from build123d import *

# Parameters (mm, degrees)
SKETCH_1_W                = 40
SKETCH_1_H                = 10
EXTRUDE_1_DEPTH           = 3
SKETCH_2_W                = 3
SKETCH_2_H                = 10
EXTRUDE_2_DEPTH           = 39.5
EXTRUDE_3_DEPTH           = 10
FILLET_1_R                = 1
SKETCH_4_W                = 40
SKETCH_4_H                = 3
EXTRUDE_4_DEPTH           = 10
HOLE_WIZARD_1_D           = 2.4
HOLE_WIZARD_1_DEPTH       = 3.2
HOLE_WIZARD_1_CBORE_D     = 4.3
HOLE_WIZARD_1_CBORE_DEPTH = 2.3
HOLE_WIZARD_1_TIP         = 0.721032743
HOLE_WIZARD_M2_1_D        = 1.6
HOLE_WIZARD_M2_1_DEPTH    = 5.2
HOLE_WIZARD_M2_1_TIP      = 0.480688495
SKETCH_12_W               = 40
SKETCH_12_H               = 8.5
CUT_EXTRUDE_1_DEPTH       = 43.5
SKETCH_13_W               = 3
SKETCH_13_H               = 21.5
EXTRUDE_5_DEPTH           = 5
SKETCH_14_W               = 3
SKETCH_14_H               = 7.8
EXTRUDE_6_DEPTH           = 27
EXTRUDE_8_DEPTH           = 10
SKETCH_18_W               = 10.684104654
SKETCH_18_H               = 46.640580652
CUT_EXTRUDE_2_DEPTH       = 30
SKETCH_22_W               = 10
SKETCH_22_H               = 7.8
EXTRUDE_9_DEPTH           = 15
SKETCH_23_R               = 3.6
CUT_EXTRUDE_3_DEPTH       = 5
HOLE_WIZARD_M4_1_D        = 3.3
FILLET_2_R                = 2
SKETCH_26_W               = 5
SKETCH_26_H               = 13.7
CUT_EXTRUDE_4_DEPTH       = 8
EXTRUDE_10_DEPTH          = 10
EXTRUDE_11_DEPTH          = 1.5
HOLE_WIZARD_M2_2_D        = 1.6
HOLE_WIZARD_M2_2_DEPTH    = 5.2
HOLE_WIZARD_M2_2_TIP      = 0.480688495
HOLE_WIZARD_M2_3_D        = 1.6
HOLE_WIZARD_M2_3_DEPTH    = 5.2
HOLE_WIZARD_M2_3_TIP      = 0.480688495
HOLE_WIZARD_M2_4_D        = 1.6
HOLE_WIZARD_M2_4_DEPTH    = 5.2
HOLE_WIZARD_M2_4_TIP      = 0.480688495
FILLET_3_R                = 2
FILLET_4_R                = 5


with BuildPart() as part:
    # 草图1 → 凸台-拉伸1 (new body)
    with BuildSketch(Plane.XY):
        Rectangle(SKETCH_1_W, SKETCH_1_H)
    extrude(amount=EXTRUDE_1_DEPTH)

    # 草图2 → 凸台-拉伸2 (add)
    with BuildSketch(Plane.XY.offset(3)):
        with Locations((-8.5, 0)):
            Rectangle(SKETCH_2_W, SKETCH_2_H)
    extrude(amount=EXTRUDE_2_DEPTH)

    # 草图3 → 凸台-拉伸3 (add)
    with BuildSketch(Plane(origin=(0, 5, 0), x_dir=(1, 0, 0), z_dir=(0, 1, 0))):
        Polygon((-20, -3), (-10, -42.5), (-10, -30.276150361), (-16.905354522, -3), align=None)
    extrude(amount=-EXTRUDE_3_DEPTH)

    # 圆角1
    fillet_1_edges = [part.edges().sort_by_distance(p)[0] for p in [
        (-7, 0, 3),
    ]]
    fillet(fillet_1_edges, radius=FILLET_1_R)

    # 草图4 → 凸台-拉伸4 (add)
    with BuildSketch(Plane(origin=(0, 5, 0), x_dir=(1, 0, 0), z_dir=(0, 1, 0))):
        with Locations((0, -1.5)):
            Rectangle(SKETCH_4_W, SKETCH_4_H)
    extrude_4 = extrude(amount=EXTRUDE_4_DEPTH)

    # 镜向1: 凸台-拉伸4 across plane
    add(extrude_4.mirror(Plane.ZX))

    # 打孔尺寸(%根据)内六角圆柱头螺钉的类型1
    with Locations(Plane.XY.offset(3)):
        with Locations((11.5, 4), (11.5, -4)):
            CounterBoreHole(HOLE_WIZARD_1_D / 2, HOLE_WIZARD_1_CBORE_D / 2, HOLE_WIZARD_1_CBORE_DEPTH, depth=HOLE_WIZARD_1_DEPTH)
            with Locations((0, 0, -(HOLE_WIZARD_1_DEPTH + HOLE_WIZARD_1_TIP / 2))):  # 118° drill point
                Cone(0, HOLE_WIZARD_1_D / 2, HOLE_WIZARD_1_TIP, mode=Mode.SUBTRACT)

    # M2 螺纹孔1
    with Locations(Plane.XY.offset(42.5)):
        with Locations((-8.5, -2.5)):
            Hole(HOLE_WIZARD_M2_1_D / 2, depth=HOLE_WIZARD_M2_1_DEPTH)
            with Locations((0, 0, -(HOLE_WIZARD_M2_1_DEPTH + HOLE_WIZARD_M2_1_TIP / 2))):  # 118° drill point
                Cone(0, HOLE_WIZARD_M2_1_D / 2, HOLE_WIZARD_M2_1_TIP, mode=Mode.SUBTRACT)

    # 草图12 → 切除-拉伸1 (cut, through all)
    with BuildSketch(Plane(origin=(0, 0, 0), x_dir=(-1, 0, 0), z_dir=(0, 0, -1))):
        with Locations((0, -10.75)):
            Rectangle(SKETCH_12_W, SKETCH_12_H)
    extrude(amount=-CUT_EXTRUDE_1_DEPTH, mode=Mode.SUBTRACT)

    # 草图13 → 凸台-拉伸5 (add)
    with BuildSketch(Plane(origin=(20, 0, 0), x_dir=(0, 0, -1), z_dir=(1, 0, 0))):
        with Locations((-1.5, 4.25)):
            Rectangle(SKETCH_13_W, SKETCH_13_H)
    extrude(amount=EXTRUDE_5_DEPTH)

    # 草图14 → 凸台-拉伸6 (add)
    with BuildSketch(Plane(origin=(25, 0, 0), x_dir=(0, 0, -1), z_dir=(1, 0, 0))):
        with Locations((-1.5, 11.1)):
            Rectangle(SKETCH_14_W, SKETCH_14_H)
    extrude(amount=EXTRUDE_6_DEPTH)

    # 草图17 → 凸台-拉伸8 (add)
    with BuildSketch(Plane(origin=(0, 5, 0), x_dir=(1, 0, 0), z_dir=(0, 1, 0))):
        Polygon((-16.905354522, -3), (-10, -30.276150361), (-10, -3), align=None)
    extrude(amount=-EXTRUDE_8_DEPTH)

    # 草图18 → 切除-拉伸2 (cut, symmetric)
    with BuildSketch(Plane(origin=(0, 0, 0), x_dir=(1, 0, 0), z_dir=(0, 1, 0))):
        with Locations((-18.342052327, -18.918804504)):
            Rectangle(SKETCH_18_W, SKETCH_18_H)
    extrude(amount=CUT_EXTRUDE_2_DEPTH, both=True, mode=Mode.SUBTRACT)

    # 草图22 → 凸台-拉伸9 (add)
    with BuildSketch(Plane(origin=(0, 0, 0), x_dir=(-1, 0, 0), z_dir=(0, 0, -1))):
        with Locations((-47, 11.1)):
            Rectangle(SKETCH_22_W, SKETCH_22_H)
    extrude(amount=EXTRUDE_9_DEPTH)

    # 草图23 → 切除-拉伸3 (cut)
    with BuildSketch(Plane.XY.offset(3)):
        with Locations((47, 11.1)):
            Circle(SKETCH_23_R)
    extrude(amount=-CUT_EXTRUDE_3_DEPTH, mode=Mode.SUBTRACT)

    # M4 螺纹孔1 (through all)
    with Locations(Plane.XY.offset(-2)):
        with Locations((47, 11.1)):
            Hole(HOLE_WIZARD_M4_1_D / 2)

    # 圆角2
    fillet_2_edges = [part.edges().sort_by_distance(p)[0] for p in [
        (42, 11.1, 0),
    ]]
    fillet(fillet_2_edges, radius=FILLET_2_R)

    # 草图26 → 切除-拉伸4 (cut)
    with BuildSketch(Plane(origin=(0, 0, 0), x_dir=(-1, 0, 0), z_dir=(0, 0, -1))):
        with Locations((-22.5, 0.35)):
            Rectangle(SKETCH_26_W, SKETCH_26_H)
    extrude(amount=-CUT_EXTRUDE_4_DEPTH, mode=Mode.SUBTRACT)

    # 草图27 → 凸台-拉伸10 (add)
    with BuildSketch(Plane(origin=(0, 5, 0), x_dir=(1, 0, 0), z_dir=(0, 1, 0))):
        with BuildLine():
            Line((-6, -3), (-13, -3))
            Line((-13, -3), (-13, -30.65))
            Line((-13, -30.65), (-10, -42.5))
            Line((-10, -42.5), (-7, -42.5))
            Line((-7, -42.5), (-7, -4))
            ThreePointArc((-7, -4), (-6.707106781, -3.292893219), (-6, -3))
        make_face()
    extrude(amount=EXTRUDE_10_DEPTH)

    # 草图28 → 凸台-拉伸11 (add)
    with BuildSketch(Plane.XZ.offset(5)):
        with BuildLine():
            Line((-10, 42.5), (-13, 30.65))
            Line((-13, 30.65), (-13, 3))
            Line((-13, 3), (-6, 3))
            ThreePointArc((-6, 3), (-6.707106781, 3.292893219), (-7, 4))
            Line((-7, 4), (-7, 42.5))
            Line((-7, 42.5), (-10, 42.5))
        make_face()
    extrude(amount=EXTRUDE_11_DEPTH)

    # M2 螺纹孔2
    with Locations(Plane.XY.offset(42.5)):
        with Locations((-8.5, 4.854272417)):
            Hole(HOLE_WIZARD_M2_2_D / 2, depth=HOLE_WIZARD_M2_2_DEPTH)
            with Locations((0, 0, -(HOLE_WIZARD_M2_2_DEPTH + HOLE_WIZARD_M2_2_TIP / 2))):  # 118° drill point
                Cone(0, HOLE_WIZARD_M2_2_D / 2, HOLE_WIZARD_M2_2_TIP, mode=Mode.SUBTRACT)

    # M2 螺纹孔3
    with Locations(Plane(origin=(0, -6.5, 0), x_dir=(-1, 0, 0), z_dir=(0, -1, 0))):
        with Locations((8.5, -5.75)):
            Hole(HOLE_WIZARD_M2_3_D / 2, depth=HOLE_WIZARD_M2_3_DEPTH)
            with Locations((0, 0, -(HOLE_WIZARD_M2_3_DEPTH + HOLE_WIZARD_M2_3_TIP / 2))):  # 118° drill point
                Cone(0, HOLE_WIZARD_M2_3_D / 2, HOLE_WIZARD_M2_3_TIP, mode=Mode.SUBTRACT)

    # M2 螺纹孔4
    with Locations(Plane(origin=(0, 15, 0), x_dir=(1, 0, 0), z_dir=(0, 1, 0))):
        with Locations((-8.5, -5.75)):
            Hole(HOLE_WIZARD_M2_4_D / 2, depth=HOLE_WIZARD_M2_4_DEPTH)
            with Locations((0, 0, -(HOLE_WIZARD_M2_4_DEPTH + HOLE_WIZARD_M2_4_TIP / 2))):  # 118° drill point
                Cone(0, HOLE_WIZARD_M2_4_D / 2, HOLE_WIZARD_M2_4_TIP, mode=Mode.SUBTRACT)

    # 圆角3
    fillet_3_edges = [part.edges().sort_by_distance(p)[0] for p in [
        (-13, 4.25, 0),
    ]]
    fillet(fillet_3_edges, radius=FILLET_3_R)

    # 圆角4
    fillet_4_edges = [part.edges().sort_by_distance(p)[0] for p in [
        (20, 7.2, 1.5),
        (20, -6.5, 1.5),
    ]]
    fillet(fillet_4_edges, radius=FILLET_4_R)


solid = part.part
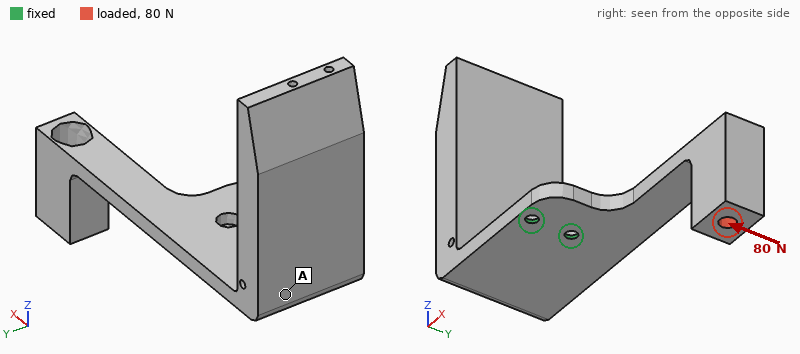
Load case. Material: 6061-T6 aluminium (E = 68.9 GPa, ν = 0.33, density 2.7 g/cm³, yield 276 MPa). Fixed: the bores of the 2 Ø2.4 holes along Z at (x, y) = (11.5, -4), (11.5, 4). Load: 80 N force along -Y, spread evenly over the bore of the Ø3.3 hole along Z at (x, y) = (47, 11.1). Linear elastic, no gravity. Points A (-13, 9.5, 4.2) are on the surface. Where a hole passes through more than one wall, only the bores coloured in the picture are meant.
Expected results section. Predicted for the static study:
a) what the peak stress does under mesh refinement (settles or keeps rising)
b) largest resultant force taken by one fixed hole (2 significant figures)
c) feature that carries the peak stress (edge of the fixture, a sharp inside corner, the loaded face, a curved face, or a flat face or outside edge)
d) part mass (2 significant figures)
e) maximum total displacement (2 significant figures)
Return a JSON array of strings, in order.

["keeps rising", "320 N", "edge of the fixture", "22 g", "0.41 mm"]
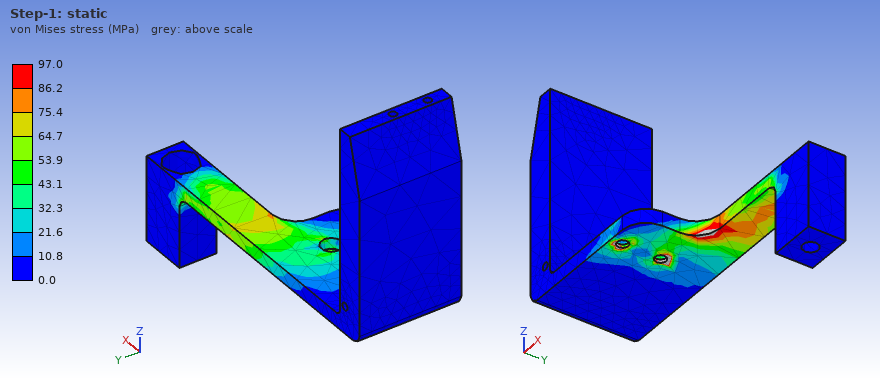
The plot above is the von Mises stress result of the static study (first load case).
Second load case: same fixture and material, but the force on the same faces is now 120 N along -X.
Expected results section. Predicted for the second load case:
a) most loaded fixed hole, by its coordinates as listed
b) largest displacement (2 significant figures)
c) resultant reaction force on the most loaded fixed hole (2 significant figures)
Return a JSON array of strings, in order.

["(11.5, 4)", "1.0 mm", "220 N"]
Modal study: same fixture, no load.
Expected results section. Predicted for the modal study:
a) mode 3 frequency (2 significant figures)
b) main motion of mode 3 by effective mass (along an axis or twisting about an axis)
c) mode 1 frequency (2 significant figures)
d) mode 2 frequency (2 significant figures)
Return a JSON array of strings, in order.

["970 Hz", "along Y", "430 Hz", "790 Hz"]
